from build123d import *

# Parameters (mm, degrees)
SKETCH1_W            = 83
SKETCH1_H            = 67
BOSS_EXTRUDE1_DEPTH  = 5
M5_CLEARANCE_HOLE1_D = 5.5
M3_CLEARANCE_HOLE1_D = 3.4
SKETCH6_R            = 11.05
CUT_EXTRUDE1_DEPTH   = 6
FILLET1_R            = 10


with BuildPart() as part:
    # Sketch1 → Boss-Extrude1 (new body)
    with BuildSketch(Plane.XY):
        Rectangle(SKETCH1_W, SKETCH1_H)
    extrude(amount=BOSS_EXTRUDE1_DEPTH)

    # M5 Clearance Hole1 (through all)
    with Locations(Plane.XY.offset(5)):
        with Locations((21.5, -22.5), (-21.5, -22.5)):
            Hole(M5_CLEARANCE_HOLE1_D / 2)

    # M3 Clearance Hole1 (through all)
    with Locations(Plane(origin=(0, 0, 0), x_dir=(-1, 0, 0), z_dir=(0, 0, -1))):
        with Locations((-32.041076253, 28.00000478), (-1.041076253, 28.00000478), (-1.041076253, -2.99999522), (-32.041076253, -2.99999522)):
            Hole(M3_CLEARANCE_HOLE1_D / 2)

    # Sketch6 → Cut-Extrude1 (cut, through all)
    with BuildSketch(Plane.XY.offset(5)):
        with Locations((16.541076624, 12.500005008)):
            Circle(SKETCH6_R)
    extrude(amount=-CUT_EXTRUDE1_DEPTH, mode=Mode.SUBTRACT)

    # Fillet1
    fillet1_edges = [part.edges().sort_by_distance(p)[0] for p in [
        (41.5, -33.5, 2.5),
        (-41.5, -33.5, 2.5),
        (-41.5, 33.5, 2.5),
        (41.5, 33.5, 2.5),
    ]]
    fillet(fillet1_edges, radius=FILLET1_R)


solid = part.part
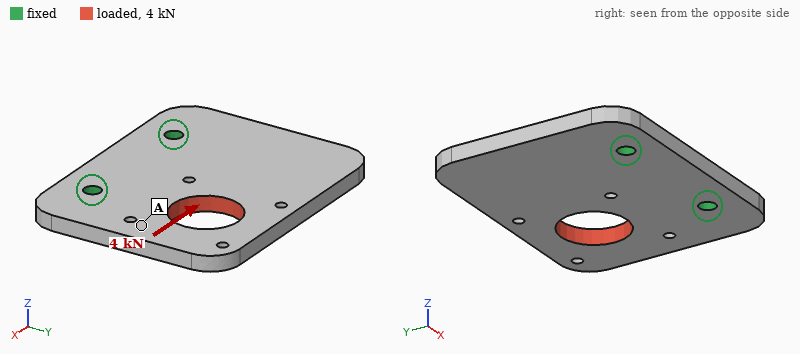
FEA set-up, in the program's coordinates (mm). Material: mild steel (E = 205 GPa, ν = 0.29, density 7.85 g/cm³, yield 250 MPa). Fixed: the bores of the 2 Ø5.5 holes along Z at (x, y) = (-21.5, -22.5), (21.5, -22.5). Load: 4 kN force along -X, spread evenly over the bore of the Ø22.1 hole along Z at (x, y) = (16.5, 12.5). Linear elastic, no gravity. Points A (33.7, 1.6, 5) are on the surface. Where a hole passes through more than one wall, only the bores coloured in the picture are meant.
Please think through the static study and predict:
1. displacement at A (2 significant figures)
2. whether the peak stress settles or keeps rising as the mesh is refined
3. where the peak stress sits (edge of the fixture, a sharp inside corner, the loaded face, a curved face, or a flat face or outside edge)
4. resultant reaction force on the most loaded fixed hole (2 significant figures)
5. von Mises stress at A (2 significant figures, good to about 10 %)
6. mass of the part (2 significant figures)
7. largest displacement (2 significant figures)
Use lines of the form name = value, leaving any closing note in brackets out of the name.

displacement at A = 10 µm
whether the peak stress settles or keeps rising as the mesh is refined = keeps rising
where the peak stress sits = edge of the fixture
resultant reaction force on the most loaded fixed hole = 3.7 kN
von Mises stress at A = 20 MPa
mass of the part = 200 g
largest displacement = 18 µm
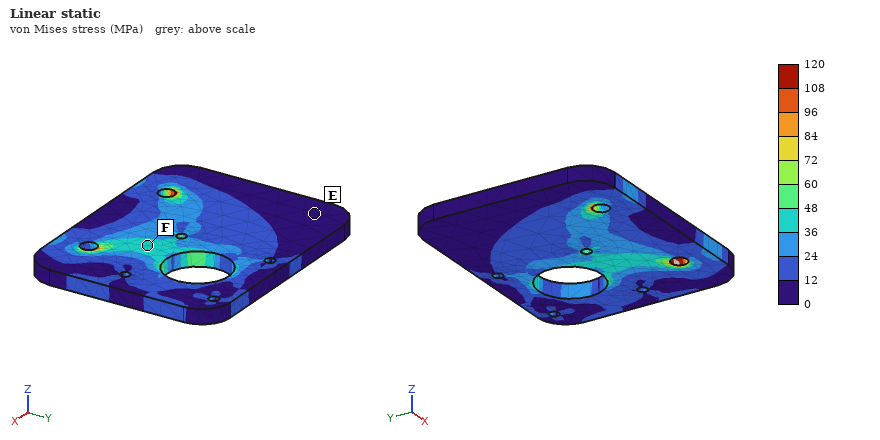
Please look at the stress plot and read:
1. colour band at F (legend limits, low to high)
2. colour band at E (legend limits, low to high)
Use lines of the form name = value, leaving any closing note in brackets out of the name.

colour band at F = 36 to 48 MPa
colour band at E = 0 to 12 MPa
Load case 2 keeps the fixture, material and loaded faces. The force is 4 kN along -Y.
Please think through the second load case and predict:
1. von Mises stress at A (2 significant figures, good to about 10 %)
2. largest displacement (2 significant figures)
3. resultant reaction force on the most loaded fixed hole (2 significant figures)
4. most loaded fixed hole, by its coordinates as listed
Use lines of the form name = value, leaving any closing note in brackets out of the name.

von Mises stress at A = 22 MPa
largest displacement = 9.0 µm
resultant reaction force on the most loaded fixed hole = 3.4 kN
most loaded fixed hole, by its coordinates as listed = (21.5, -22.5)
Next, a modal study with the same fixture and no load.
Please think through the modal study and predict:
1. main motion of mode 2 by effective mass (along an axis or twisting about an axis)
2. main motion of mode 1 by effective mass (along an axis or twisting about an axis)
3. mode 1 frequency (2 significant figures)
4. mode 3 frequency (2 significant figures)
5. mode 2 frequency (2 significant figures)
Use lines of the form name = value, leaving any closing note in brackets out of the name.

main motion of mode 2 by effective mass = twisting about Y
main motion of mode 1 by effective mass = along Z
mode 1 frequency = 1300 Hz
mode 3 frequency = 4700 Hz
mode 2 frequency = 2300 Hz
